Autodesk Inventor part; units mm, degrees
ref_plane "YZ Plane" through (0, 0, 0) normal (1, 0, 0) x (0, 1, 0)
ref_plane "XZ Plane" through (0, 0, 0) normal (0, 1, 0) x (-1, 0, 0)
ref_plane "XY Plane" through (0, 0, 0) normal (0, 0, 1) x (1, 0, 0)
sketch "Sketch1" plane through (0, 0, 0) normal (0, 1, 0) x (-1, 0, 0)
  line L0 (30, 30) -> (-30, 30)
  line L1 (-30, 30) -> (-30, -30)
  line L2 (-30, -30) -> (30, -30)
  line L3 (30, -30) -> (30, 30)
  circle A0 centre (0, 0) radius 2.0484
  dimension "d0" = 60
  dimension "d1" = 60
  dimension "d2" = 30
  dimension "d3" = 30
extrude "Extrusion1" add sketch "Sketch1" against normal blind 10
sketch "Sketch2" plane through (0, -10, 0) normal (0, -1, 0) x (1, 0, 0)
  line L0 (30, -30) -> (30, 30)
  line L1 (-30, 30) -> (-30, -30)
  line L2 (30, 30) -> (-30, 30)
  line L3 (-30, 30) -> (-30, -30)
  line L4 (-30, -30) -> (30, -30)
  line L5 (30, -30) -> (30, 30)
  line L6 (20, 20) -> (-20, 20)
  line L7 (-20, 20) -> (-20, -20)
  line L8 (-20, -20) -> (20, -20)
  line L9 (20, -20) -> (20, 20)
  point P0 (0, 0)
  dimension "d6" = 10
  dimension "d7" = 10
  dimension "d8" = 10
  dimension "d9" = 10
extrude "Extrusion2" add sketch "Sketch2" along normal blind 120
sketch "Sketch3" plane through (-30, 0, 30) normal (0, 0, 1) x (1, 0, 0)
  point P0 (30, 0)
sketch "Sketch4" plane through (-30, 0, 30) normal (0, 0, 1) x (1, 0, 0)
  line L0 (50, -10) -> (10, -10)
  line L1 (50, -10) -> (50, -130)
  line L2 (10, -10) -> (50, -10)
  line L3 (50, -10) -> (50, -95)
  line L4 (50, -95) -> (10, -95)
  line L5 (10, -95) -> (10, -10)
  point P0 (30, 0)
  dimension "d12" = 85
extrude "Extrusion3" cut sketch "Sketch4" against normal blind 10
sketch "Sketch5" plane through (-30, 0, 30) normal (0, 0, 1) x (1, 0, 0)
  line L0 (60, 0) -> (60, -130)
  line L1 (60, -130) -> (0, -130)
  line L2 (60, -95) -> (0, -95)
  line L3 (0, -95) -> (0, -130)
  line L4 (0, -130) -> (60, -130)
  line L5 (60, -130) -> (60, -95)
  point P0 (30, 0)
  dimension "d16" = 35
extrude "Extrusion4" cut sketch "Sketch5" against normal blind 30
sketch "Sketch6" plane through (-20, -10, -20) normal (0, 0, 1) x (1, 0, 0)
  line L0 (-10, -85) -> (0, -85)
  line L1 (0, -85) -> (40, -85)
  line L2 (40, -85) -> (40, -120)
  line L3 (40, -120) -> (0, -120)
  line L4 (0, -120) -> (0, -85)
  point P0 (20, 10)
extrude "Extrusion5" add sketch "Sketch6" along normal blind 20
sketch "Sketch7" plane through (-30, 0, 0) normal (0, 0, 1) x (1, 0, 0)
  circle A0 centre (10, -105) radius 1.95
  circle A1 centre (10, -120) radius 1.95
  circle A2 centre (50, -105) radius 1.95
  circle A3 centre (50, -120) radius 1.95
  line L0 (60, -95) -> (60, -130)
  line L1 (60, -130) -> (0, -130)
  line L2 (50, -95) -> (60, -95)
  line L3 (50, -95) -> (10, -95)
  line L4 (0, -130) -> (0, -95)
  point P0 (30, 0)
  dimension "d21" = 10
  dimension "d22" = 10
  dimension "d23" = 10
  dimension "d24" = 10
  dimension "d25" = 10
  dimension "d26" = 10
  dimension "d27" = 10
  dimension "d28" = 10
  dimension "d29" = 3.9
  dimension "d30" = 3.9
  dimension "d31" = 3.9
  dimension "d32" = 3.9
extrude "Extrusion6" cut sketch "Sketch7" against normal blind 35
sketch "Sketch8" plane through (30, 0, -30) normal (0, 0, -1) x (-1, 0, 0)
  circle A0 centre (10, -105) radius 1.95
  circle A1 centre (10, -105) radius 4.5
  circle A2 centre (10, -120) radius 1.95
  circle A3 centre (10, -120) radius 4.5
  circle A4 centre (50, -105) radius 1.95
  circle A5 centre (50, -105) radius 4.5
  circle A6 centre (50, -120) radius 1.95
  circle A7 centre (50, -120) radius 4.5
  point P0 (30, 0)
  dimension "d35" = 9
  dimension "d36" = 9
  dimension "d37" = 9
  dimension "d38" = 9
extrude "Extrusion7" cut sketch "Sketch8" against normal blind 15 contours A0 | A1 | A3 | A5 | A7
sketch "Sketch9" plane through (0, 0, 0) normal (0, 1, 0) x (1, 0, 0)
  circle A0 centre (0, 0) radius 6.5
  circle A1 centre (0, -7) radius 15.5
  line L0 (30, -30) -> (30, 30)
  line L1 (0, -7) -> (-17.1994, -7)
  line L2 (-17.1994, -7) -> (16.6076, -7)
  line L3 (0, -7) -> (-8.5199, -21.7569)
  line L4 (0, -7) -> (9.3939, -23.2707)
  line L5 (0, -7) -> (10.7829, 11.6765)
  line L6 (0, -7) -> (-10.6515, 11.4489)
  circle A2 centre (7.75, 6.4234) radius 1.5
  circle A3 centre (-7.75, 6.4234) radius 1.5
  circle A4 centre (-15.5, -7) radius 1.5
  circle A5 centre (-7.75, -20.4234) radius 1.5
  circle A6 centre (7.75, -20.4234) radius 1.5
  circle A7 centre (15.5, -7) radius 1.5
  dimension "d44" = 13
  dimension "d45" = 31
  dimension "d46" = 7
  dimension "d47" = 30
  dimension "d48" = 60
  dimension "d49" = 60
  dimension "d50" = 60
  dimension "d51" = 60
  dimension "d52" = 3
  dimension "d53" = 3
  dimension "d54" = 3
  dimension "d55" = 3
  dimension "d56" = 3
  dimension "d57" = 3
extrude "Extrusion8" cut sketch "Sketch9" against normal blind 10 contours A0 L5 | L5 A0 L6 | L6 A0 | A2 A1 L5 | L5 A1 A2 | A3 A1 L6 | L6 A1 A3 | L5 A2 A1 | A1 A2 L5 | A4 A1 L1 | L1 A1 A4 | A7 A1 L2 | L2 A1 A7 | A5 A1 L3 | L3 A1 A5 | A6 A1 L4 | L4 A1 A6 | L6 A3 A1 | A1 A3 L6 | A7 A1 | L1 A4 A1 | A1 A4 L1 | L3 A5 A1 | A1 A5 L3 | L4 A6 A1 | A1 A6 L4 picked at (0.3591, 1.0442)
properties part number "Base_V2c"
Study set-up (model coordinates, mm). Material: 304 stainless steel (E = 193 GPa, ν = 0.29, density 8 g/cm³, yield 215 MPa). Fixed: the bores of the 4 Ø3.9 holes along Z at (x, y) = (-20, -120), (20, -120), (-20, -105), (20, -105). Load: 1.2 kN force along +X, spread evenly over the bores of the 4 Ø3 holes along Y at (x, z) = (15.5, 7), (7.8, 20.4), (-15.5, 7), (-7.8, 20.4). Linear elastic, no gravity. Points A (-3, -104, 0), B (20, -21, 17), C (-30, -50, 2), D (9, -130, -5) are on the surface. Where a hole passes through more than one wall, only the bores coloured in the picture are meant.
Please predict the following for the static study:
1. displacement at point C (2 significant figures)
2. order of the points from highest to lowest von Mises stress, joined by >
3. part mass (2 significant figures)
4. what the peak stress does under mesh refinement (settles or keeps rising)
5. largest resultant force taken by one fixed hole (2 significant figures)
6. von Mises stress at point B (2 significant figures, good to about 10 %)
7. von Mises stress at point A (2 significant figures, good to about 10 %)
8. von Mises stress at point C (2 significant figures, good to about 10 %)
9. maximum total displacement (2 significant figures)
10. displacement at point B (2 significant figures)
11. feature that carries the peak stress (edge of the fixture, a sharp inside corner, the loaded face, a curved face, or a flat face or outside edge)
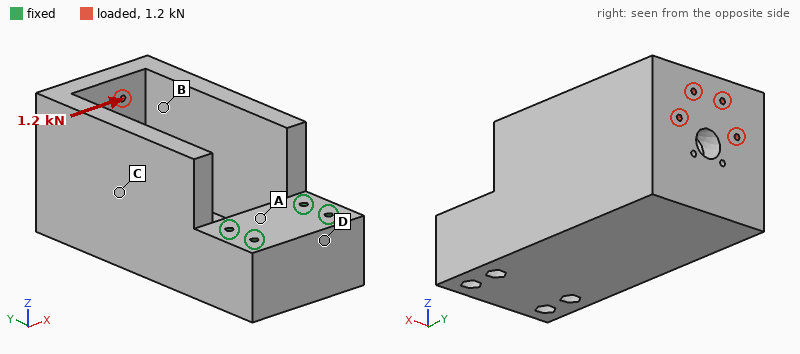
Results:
20 µm
B > C > A > D
1.8 kg
keeps rising
2.0 kN
12 MPa
5.9 MPa
9.4 MPa
49 µm
36 µm
edge of the fixture
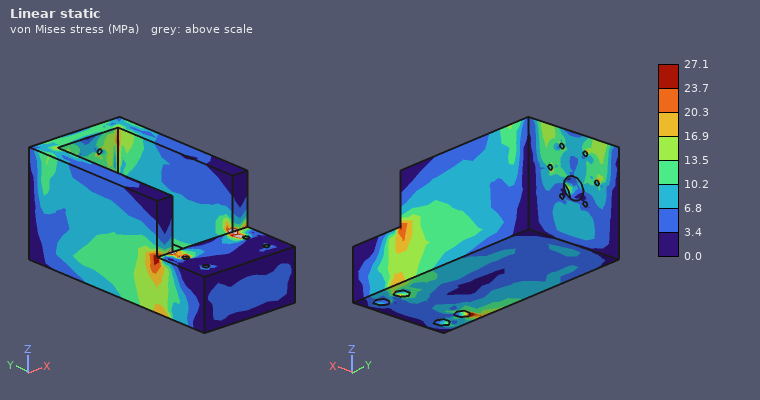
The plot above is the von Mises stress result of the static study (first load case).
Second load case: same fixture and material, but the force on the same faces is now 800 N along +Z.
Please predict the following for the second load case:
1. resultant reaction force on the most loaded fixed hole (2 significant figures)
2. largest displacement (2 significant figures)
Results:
1.8 kN
27 µm
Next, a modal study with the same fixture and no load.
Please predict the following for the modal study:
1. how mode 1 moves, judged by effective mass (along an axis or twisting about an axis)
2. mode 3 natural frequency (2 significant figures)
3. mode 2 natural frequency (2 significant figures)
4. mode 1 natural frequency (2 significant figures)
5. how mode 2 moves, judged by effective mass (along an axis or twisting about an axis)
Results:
along Z
3300 Hz
1300 Hz
1100 Hz
along X
